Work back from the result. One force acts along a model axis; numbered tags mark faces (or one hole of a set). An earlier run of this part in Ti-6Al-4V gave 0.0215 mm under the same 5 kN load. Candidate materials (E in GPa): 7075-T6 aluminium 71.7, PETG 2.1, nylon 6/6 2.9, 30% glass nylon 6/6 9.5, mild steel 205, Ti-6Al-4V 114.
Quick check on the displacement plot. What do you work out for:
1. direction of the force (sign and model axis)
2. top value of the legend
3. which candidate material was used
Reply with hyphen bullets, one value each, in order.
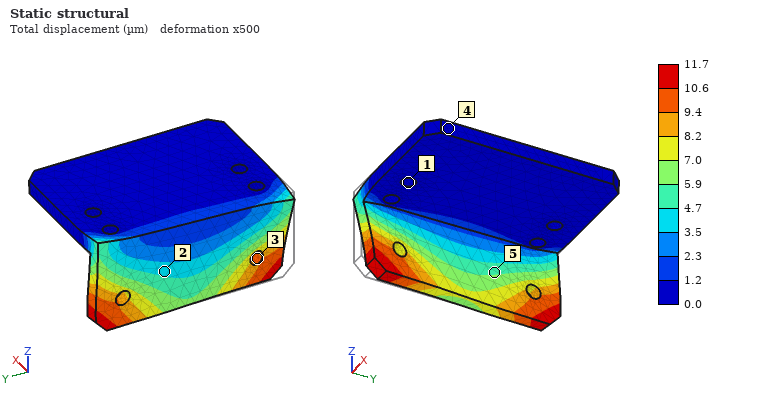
- +Y
- 11.7 µm
- mild steel
